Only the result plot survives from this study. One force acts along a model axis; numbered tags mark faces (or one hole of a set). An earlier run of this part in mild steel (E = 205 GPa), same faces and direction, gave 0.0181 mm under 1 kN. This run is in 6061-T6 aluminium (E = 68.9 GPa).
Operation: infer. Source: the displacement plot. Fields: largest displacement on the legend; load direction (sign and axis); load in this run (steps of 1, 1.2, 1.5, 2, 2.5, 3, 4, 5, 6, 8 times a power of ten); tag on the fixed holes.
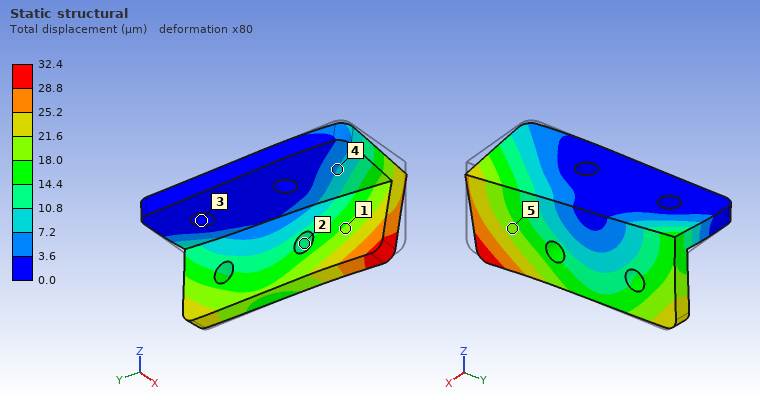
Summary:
32.4 µm
+Y
600 N
3
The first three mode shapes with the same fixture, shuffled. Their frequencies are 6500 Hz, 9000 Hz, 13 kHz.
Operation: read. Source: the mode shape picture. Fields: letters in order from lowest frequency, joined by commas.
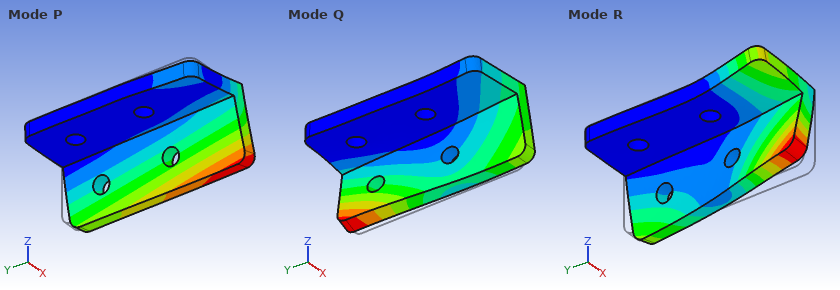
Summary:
P, Q, R
